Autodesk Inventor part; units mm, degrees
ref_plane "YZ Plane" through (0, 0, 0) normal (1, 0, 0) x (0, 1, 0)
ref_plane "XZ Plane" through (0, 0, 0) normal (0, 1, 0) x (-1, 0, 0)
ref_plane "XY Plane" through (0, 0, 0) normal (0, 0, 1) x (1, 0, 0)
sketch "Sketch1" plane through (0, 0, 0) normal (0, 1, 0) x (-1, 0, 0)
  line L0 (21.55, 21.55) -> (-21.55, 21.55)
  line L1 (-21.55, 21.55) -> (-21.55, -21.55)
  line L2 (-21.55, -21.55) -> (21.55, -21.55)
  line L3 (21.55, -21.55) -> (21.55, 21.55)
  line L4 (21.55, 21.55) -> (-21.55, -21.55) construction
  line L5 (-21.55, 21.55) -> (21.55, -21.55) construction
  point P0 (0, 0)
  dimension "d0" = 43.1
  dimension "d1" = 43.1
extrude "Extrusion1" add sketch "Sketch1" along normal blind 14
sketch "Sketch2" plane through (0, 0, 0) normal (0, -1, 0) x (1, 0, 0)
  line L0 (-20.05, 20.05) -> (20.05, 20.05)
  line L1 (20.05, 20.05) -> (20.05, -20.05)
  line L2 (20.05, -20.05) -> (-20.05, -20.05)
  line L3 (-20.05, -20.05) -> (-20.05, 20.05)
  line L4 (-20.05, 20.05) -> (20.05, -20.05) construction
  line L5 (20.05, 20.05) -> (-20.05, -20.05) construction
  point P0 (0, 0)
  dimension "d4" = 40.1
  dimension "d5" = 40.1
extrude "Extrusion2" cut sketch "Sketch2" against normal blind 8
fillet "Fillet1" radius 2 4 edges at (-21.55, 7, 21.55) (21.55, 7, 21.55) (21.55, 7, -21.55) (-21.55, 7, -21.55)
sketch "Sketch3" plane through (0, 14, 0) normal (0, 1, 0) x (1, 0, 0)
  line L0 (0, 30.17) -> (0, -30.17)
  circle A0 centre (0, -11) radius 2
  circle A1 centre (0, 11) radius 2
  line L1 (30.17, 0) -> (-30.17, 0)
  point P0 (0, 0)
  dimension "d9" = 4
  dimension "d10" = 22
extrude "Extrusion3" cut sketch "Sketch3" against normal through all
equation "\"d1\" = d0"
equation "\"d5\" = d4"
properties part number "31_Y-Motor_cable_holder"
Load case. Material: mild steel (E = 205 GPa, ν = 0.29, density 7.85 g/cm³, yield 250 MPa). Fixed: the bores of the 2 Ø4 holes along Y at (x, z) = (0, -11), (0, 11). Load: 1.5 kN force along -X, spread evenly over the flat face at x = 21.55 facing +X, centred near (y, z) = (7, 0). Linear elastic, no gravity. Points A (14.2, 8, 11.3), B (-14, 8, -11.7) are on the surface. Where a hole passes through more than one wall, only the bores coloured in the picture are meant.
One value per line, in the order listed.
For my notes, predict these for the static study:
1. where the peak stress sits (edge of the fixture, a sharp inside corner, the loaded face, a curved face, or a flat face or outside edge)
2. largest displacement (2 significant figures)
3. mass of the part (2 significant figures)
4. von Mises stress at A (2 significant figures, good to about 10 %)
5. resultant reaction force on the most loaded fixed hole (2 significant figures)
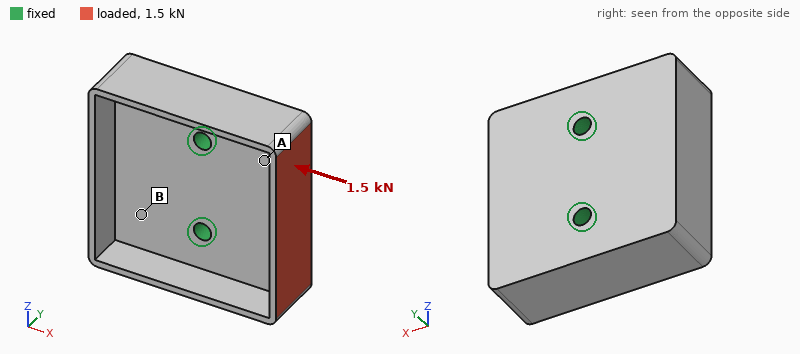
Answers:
the loaded face
38 µm
100 g
21 MPa
770 N
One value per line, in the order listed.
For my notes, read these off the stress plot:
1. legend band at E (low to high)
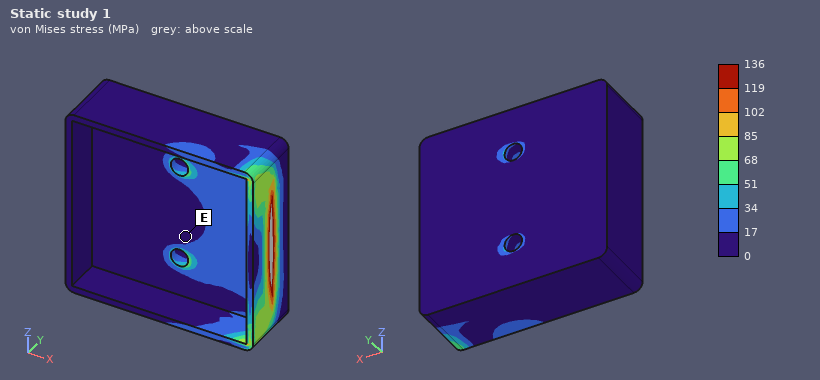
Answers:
0 to 17 MPa
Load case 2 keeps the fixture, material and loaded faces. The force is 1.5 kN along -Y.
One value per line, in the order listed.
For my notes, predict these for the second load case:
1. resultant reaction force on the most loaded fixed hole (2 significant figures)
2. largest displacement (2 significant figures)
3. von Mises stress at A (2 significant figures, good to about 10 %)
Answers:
770 N
42 µm
28 MPa
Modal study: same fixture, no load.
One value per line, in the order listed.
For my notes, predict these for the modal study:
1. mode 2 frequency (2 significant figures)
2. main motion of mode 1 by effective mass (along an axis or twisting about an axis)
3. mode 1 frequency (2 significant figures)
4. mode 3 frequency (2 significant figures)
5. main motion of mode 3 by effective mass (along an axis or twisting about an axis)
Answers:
10 kHz
twisting about Z
7200 Hz
11 kHz
along Y
